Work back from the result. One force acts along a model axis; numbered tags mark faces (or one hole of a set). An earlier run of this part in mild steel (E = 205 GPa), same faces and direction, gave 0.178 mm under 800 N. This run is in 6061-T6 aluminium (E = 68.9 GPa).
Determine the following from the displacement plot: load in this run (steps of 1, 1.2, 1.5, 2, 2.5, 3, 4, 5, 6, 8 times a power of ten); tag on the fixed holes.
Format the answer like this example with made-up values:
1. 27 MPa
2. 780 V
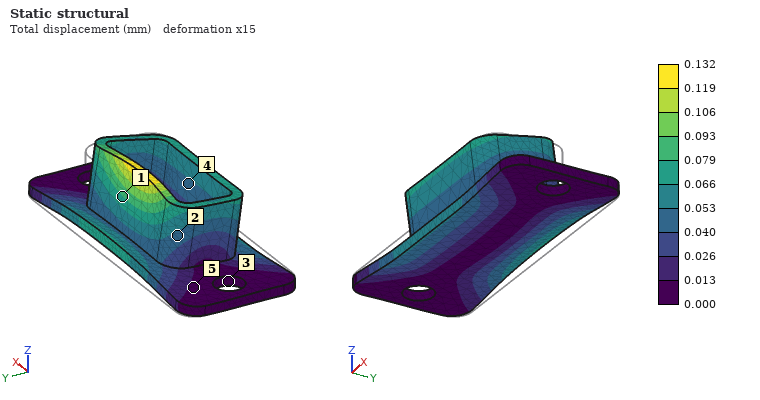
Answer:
1. 200 N
2. 3
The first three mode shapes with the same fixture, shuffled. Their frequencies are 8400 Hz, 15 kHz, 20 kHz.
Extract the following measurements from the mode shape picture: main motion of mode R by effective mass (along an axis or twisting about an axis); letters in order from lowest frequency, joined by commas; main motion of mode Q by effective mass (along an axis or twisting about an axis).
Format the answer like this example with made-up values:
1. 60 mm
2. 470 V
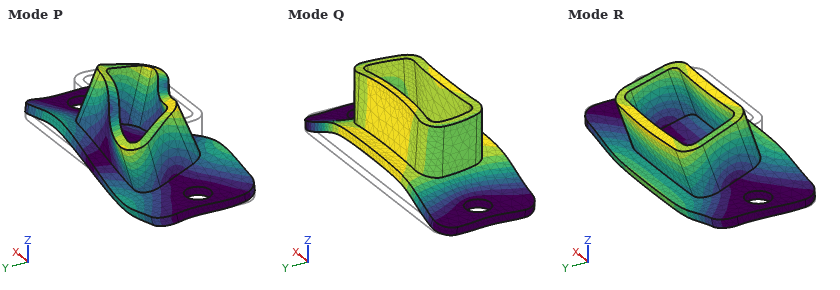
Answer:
1. along Y
2. R, Q, P
3. along Z
